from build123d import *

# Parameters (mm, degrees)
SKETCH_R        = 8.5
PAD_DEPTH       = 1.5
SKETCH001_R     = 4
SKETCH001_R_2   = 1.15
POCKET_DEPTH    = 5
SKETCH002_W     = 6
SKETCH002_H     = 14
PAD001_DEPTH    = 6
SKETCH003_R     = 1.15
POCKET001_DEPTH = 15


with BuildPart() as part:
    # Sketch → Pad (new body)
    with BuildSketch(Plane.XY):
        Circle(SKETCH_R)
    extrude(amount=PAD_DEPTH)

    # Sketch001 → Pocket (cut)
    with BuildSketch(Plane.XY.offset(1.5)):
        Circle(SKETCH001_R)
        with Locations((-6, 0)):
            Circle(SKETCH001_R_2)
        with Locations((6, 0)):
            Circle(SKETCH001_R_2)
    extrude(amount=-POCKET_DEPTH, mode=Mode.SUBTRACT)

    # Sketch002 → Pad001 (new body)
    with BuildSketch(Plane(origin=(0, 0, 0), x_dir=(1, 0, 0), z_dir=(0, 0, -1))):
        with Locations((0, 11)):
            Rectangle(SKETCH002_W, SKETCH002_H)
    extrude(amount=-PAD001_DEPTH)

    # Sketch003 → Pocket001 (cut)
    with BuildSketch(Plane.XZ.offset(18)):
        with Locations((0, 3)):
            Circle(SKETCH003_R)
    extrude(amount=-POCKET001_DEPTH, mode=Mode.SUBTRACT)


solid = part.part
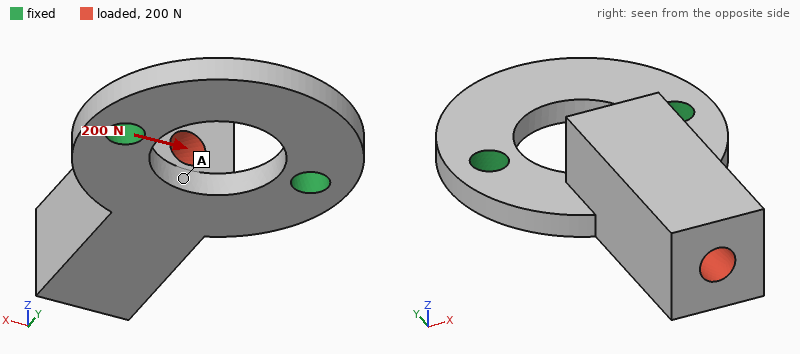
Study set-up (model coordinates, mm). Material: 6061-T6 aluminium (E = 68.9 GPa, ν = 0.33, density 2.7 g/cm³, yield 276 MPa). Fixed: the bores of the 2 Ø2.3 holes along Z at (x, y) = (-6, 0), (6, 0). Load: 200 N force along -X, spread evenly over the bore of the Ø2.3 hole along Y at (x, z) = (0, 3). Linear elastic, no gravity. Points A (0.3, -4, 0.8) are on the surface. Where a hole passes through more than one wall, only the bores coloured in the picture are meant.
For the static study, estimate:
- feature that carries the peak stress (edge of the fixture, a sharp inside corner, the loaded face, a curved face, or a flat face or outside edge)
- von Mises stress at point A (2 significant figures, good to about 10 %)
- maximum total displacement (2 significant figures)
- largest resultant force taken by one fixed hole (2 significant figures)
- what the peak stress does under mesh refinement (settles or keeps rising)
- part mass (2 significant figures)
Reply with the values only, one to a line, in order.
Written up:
edge of the fixture
18 MPa
31 µm
190 N
keeps rising
1.8 g
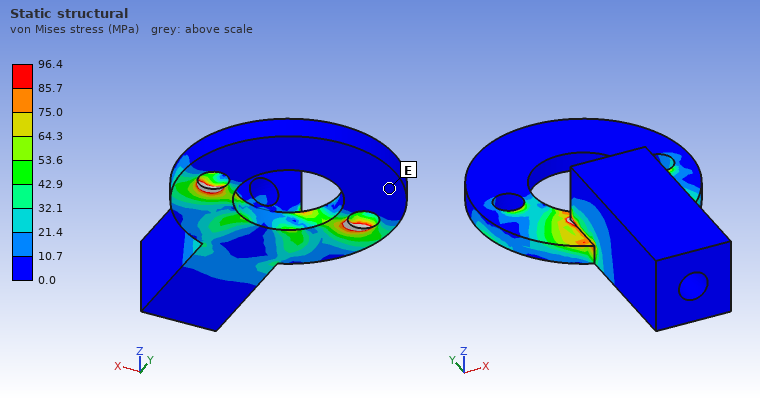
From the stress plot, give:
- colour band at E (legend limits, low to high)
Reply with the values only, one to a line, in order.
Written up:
0.0 to 10.7 MPa
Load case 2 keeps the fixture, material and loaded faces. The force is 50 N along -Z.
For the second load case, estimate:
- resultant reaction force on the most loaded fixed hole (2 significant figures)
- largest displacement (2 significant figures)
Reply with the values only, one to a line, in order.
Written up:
25 N
0.19 mm
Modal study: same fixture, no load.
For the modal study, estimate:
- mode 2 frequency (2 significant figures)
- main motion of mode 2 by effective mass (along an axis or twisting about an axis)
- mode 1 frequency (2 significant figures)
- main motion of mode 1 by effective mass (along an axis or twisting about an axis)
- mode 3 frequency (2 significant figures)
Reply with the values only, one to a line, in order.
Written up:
14 kHz
along X
2800 Hz
along Z
18 kHz
